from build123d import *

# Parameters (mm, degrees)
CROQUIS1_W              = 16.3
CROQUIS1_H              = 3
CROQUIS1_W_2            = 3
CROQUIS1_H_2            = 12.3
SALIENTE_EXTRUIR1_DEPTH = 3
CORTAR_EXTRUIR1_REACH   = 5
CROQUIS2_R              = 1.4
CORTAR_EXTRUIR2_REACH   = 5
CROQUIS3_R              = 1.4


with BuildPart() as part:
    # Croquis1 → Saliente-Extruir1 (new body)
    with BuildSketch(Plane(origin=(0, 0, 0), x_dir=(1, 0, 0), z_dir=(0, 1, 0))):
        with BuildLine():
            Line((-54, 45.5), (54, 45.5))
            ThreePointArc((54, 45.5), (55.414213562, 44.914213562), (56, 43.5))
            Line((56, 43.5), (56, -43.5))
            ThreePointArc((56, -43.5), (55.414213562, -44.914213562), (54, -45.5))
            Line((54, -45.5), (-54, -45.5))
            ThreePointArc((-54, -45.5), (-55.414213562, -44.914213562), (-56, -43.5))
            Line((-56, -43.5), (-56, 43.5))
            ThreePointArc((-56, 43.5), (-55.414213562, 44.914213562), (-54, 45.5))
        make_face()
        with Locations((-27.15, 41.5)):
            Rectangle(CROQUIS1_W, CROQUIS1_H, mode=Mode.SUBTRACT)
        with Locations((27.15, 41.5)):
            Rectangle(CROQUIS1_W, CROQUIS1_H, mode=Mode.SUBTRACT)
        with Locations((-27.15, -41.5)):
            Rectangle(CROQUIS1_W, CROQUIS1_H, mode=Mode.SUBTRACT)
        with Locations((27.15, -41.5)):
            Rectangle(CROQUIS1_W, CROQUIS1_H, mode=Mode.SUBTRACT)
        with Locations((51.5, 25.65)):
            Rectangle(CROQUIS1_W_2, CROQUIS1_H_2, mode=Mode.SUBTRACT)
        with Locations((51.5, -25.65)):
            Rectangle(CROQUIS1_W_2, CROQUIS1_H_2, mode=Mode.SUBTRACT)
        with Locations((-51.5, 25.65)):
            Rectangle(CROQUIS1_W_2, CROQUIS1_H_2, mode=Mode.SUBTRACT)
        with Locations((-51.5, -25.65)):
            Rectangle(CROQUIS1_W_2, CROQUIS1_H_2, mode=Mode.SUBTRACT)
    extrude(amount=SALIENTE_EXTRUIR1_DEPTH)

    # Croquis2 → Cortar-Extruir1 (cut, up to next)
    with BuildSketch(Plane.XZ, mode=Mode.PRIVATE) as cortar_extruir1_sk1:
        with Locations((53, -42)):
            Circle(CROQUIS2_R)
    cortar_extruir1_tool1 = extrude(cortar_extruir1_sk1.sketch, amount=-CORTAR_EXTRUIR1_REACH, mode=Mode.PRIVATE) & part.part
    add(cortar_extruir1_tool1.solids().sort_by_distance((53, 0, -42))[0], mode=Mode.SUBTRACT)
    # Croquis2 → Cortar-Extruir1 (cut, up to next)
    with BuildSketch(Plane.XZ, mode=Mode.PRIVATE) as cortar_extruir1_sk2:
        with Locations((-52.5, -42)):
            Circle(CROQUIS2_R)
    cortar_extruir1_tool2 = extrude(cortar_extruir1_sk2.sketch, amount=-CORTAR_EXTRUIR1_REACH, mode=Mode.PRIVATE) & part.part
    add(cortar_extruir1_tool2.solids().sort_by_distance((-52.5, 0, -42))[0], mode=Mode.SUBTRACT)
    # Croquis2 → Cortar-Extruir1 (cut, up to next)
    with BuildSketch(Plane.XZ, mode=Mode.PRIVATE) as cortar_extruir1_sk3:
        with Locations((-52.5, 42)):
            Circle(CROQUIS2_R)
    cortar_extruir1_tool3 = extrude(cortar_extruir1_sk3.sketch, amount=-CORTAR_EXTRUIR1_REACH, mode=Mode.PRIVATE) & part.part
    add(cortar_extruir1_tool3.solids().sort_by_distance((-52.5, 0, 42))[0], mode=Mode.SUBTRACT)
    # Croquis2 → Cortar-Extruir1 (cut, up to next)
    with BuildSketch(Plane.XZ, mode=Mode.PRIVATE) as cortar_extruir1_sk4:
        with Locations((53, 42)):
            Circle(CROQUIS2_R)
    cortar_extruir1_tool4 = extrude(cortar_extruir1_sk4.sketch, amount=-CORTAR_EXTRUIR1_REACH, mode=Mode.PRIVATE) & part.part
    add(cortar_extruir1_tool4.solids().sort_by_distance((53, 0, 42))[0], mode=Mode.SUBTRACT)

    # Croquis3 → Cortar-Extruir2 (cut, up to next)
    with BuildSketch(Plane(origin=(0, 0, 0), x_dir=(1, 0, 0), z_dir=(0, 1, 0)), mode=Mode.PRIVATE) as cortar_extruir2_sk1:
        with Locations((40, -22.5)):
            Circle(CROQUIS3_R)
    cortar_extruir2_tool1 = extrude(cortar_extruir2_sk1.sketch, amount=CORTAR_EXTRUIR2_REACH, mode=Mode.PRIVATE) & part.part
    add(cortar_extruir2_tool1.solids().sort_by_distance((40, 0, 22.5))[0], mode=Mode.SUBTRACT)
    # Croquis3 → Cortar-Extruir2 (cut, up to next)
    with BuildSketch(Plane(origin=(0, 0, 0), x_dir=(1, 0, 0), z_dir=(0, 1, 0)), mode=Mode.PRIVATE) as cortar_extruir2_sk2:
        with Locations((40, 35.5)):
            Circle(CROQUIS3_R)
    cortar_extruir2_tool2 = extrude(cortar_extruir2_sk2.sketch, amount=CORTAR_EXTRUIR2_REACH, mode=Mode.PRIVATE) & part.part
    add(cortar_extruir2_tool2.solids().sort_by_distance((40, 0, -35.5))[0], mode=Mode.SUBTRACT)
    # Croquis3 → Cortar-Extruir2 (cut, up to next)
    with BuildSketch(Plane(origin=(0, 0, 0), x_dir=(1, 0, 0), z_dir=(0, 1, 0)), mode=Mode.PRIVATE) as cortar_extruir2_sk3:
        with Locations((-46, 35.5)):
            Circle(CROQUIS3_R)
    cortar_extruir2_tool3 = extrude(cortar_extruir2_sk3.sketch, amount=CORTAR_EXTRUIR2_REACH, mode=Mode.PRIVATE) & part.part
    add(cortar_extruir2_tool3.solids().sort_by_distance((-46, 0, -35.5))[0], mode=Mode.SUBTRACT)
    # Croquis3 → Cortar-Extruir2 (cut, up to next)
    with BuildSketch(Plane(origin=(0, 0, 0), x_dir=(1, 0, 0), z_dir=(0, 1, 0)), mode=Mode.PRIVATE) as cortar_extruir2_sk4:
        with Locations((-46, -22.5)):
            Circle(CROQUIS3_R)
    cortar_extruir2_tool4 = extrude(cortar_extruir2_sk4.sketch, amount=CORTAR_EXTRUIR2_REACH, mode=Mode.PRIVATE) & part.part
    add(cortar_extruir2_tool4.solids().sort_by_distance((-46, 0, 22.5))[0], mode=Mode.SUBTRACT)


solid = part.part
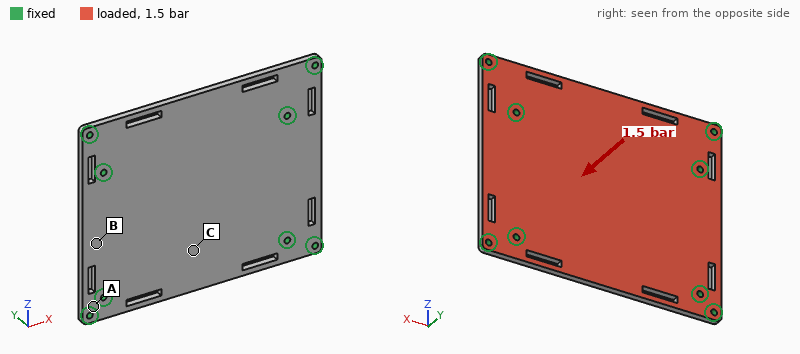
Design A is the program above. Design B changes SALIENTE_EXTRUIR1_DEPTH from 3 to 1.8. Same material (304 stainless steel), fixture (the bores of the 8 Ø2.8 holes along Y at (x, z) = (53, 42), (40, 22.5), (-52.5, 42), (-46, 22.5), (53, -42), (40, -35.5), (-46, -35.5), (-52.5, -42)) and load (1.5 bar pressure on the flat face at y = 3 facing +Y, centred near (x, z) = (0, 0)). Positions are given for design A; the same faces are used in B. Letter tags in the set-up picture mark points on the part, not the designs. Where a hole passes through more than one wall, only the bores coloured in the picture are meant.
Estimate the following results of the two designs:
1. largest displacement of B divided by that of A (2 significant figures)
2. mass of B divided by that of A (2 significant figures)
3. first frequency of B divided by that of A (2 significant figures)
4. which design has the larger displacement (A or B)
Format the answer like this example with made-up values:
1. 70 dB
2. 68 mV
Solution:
1. 4.4
2. 0.60
3. 0.62
4. B
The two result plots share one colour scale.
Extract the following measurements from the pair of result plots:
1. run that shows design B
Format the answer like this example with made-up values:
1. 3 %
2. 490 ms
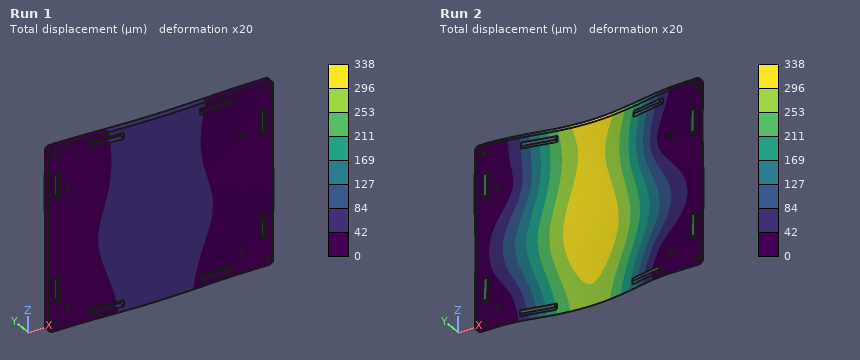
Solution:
1. Run 2
